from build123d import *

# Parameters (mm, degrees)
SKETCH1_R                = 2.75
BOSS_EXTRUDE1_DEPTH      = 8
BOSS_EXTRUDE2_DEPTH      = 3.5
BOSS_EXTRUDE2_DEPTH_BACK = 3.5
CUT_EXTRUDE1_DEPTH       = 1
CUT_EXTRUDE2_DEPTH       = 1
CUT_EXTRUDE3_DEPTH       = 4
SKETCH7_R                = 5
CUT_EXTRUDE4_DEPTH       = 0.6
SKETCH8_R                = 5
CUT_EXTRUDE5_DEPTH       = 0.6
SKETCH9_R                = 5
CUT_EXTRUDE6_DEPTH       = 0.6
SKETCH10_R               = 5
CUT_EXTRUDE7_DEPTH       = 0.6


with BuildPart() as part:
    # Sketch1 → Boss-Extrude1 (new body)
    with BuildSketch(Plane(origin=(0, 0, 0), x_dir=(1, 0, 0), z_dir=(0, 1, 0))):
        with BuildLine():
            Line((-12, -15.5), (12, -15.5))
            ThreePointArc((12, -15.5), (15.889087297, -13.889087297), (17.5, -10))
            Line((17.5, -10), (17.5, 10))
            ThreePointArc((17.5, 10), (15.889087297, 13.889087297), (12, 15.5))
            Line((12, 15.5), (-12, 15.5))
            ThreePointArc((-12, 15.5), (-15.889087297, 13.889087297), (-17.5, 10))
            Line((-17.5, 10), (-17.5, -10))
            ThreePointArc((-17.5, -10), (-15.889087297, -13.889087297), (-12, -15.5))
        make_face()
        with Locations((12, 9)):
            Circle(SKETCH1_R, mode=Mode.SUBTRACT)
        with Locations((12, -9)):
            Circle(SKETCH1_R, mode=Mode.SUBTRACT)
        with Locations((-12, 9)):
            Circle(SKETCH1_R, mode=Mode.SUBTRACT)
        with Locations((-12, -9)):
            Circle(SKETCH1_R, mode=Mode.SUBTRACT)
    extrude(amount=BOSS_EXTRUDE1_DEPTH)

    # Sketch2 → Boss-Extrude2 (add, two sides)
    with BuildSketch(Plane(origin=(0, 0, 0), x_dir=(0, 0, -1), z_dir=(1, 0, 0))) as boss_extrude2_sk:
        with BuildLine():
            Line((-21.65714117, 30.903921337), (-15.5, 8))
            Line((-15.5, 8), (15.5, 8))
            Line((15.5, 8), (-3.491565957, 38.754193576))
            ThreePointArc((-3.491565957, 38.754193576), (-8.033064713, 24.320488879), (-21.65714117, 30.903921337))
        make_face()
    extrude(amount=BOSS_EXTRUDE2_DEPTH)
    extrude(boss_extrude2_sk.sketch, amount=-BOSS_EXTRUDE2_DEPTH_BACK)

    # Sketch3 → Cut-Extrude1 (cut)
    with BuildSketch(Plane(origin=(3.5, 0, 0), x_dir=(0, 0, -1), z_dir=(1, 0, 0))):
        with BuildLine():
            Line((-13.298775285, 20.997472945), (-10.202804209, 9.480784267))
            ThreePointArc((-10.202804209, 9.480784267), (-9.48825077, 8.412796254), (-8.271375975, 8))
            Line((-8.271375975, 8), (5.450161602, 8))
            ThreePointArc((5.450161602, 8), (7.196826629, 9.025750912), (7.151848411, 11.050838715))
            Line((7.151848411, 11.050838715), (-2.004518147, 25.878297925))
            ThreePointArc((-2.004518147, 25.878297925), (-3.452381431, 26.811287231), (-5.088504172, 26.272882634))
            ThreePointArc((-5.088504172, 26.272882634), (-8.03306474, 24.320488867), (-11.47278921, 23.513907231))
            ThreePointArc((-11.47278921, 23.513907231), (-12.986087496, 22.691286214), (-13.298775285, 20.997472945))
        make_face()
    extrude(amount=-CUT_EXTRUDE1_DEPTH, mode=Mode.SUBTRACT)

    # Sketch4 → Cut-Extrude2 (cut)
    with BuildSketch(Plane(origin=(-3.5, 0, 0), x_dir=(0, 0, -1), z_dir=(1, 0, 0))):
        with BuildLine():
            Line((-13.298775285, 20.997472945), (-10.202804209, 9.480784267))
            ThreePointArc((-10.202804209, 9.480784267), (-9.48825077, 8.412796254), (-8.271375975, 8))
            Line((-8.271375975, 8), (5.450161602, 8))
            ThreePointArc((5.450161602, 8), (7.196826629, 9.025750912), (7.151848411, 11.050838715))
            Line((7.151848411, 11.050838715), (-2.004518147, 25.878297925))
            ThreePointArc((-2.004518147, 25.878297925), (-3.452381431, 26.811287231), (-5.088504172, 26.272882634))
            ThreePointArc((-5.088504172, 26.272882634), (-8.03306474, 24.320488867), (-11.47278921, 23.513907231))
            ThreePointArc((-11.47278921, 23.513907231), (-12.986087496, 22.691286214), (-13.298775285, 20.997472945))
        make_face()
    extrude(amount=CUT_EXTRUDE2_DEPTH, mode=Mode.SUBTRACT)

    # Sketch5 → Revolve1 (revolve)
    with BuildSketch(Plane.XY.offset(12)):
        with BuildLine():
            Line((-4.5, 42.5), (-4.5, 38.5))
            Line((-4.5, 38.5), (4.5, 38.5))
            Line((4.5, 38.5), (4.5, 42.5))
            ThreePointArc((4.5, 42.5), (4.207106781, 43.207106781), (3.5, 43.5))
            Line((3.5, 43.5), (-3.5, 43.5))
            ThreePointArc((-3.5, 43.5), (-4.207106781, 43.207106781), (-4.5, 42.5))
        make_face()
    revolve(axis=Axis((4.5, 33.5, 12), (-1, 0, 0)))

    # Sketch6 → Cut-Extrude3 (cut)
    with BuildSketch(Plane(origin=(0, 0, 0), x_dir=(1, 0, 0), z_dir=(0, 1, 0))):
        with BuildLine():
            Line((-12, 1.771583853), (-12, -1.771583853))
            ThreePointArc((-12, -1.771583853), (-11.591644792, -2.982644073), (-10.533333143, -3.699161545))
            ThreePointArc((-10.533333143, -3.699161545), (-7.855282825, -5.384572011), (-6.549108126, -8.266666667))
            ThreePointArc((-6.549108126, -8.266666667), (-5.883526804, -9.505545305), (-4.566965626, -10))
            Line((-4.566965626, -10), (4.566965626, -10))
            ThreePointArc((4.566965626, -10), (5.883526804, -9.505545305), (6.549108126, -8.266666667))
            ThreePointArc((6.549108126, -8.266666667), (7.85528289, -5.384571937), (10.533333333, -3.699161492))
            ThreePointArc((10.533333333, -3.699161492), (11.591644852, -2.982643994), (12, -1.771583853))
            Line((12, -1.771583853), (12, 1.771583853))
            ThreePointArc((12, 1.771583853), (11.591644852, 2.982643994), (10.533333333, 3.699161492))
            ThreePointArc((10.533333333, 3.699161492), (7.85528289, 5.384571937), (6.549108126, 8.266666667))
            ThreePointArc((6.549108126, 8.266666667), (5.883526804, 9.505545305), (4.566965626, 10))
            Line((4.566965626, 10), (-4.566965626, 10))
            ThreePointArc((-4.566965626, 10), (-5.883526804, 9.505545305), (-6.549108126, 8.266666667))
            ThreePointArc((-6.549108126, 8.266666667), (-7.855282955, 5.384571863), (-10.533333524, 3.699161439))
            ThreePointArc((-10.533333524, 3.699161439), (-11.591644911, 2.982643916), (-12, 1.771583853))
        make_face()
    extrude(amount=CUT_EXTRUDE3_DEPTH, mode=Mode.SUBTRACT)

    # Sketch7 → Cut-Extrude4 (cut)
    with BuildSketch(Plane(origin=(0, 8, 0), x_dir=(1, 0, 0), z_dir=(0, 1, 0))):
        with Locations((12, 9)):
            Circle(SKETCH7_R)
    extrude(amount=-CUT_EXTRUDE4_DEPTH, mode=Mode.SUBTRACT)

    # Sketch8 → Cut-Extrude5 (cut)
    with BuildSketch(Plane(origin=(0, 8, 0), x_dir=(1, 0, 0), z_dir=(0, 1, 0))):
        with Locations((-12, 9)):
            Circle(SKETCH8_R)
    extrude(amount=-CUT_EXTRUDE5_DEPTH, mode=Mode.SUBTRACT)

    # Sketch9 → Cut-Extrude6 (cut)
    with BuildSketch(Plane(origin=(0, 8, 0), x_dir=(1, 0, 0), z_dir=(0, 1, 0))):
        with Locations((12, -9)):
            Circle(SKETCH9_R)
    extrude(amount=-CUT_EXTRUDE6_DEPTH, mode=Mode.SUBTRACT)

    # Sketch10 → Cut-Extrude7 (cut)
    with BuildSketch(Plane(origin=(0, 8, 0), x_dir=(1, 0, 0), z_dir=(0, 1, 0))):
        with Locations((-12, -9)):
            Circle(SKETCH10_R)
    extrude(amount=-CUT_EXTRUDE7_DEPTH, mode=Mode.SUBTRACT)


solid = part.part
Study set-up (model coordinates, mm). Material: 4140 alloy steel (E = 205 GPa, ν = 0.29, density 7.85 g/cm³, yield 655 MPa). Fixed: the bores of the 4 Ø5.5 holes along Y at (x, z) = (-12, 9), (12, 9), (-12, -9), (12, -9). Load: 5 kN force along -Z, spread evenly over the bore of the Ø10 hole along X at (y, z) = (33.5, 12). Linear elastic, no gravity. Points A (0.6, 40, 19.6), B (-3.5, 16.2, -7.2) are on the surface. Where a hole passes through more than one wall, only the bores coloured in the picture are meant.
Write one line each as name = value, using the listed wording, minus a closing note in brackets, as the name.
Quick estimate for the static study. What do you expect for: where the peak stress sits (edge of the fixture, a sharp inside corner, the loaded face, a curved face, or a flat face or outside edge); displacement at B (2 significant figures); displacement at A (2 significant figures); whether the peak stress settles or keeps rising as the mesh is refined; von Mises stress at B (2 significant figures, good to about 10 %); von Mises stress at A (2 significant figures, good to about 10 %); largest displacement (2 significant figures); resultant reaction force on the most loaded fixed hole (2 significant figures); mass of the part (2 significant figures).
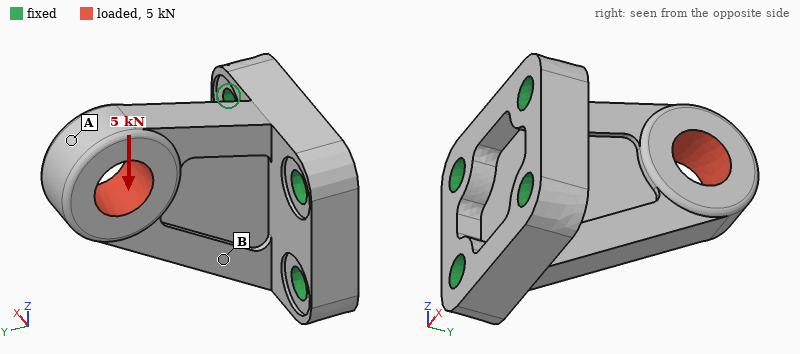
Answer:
where the peak stress sits = edge of the fixture
displacement at B = 17 µm
displacement at A = 74 µm
whether the peak stress settles or keeps rising as the mesh is refined = keeps rising
von Mises stress at B = 110 MPa
von Mises stress at A = 46 MPa
largest displacement = 75 µm
resultant reaction force on the most loaded fixed hole = 3.6 kN
mass of the part = 89 g
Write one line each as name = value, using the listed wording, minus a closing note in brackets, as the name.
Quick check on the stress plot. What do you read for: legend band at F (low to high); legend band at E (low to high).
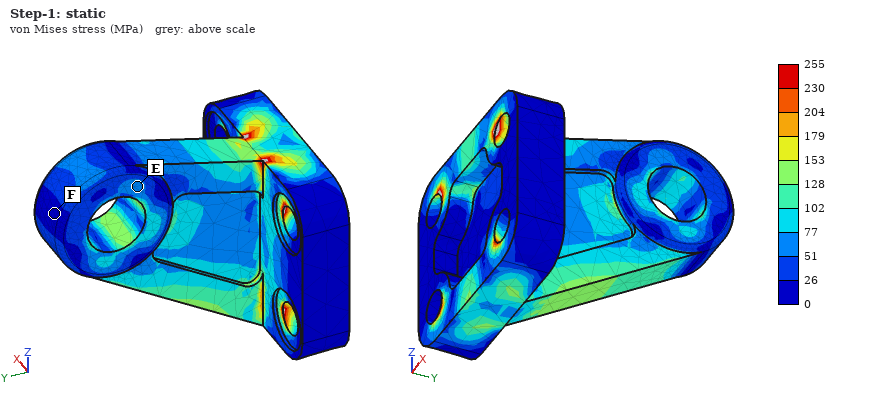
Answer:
legend band at F = 0 to 26 MPa
legend band at E = 51 to 77 MPa
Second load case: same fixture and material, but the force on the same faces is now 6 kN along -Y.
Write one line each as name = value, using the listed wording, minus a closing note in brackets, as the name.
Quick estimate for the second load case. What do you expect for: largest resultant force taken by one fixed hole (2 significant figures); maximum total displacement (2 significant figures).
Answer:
largest resultant force taken by one fixed hole = 3.2 kN
maximum total displacement = 37 µm
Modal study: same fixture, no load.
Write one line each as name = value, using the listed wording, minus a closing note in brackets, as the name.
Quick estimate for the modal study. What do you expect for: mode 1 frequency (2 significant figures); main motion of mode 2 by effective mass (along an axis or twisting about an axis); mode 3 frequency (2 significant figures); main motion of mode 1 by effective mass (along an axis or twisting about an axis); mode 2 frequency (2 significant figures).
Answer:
mode 1 frequency = 3800 Hz
main motion of mode 2 by effective mass = along Z
mode 3 frequency = 12 kHz
main motion of mode 1 by effective mass = along X
mode 2 frequency = 9700 Hz
